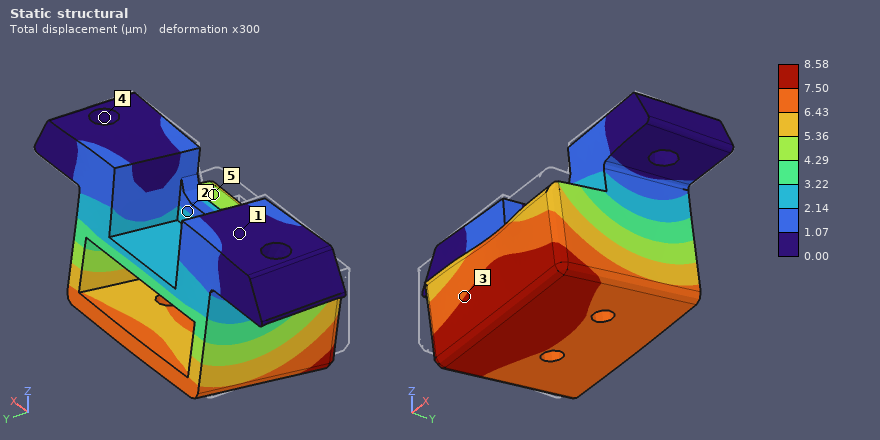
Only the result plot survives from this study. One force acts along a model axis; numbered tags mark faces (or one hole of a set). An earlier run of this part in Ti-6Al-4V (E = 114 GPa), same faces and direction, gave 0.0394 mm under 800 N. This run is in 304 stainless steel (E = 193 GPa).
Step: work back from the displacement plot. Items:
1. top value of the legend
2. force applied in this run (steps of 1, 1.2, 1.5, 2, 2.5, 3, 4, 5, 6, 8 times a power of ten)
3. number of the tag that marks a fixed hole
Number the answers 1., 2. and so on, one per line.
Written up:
1. 8.58 µm
2. 300 N
3. 4
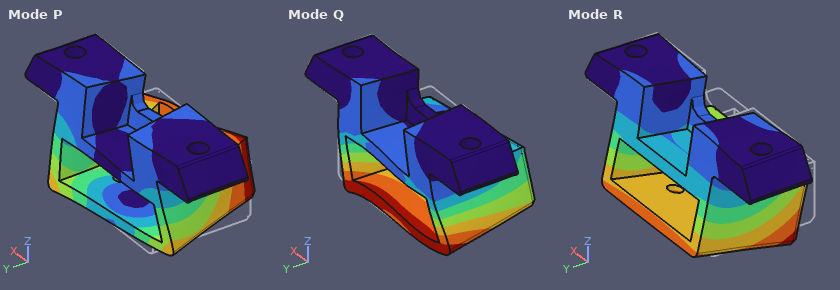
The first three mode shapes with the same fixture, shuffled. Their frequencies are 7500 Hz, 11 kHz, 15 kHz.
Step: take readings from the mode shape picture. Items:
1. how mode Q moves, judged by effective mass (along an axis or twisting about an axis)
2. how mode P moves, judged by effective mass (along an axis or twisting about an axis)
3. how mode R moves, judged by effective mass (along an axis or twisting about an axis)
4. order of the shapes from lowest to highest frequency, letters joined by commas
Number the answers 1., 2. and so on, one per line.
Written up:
1. along X
2. along X
3. along Y
4. R, Q, P
